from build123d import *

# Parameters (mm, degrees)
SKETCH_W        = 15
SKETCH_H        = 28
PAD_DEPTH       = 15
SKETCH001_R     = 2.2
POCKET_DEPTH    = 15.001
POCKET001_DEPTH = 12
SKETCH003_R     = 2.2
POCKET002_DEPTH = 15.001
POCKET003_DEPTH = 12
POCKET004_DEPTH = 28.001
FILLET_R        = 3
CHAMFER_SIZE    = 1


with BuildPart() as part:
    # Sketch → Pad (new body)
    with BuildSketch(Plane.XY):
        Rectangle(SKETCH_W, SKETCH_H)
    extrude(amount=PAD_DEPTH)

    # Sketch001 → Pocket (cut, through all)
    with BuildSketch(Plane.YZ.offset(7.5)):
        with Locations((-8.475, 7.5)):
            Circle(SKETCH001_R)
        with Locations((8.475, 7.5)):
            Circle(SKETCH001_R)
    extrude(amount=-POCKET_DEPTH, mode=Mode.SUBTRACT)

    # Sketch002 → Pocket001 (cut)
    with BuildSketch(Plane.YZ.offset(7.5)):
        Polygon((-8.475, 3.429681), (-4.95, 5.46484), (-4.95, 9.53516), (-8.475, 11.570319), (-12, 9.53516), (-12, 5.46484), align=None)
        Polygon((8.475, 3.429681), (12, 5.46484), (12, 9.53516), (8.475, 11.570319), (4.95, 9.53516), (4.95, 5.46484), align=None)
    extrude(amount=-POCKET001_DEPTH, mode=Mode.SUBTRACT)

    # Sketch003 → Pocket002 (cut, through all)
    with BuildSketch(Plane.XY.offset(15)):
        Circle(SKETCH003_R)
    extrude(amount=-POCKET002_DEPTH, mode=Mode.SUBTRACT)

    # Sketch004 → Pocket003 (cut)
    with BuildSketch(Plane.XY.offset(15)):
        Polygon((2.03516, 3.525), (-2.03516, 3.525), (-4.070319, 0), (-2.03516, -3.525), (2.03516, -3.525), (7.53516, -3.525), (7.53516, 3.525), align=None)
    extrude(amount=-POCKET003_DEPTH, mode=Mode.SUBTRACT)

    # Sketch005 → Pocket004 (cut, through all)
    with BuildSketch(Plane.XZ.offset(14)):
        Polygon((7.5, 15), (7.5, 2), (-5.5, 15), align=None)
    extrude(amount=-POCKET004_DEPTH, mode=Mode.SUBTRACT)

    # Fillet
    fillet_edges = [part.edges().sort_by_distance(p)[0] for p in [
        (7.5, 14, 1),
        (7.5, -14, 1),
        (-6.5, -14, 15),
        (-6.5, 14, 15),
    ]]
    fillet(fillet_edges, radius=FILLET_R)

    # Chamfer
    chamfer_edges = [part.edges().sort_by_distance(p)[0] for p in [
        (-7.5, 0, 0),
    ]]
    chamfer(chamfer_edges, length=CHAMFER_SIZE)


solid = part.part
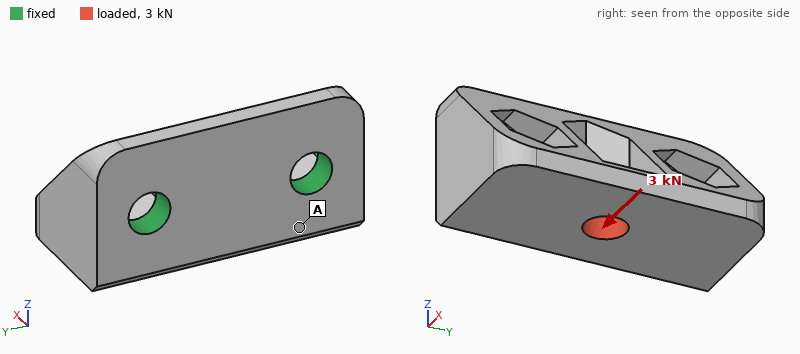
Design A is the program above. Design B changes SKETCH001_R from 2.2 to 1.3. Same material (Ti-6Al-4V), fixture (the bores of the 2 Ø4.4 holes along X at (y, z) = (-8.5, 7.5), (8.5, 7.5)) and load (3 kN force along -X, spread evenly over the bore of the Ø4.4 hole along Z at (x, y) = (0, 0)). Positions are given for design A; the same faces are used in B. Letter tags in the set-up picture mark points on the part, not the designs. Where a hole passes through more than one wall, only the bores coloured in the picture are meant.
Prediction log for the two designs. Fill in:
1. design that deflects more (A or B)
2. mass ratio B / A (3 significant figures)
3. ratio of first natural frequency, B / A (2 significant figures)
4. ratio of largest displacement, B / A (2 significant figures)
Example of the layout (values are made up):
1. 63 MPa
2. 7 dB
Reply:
1. B
2. 1.02
3. 0.72
4. 1.8
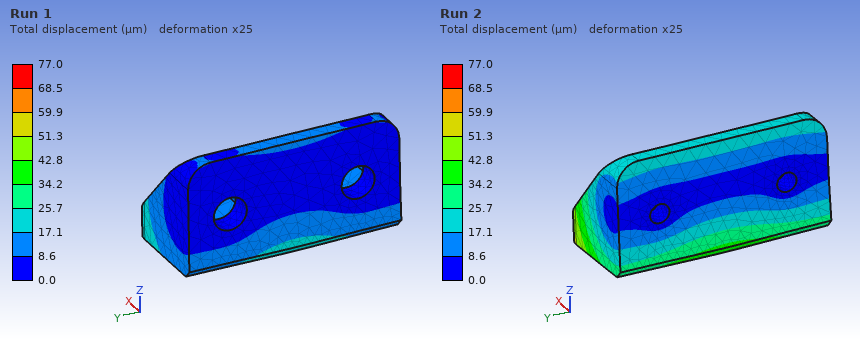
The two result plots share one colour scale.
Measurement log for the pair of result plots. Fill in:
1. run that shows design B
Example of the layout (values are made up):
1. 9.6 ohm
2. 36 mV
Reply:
1. Run 2
